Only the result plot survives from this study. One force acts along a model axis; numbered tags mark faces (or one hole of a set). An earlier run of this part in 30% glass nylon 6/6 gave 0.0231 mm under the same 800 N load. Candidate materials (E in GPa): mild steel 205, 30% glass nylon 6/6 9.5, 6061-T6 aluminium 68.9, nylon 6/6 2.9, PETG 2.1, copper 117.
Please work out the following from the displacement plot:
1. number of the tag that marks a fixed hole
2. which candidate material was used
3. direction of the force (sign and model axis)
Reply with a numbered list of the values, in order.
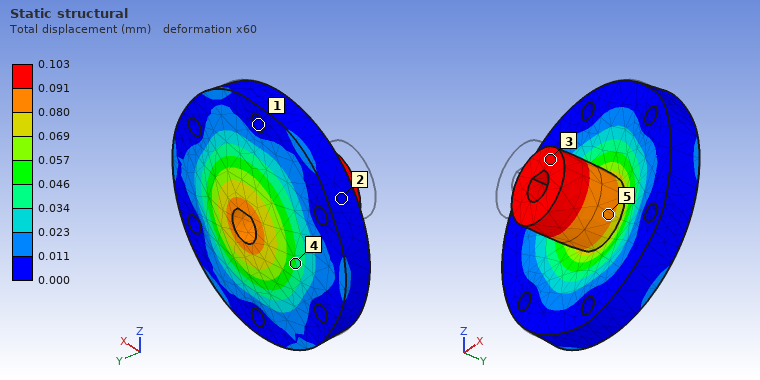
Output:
1. 1
2. PETG
3. +Y
